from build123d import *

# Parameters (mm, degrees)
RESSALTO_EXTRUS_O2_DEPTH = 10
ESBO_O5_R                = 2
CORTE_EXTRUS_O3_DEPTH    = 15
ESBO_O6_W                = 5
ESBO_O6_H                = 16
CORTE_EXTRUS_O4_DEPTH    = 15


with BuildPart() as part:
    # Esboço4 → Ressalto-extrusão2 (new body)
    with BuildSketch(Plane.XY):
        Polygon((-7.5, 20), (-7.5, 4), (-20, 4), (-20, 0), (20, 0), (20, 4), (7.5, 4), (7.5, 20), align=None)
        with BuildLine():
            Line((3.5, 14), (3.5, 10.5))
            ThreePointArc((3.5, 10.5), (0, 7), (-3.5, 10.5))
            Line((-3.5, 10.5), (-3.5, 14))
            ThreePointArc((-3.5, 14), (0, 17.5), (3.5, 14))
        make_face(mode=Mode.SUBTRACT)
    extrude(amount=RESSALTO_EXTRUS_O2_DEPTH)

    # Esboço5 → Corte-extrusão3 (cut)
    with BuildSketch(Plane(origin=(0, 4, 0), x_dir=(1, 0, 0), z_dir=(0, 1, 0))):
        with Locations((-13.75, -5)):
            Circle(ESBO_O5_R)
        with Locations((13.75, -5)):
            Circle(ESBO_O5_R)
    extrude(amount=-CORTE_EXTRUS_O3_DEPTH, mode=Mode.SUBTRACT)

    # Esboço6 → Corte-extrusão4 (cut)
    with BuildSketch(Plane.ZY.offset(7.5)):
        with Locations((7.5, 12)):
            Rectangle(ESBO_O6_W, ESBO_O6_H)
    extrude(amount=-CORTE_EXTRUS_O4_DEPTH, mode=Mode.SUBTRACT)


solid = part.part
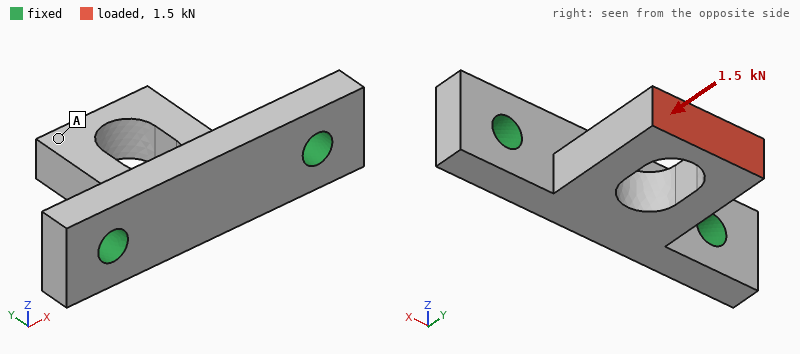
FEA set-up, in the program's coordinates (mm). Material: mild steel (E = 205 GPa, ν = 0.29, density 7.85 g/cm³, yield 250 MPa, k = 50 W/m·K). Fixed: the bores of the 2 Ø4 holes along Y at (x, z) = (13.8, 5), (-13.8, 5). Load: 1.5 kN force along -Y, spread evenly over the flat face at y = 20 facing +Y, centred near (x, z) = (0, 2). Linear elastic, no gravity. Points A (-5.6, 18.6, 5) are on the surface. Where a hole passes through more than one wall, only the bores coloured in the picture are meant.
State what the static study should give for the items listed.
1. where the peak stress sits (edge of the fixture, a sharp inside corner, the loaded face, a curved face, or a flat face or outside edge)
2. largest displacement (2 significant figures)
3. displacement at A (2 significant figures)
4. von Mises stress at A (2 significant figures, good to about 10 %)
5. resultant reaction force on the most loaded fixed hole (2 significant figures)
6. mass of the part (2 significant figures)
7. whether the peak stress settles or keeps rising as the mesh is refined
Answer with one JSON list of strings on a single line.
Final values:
["edge of the fixture", "18 µm", "14 µm", "24 MPa", "780 N", "19 g", "keeps rising"]
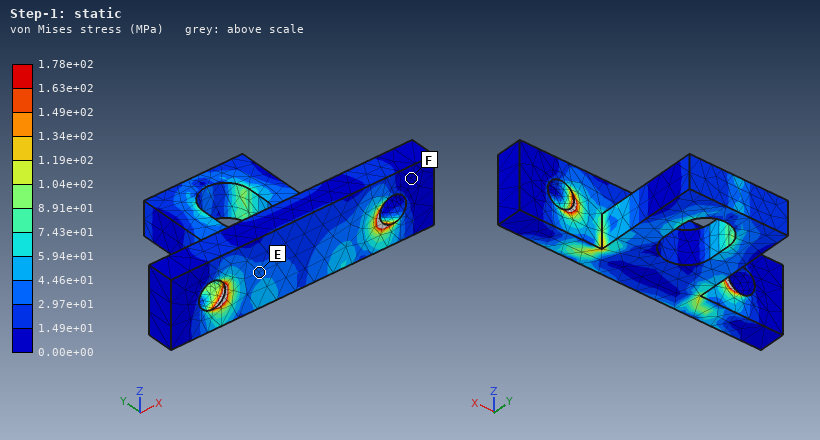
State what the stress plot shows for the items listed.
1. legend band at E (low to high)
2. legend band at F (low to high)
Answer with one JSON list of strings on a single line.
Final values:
["2.97e+01 to 4.46e+01 MPa", "0.00e+00 to 1.49e+01 MPa"]
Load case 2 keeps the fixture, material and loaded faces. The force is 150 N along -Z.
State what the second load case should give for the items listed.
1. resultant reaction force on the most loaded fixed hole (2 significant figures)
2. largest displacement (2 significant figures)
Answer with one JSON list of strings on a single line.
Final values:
["76 N", "26 µm"]
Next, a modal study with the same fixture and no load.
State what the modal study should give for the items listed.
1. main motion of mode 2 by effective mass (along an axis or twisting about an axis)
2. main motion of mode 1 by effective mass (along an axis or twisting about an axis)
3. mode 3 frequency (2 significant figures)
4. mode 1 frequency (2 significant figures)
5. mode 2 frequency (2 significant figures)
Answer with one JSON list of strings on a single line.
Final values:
["along X", "along Z", "22 kHz", "7900 Hz", "17 kHz"]
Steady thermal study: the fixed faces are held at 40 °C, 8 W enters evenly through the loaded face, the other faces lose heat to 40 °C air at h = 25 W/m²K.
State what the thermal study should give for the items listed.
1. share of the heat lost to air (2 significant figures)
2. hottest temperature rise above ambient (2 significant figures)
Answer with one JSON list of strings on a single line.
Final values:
["10 %", "70 K"]
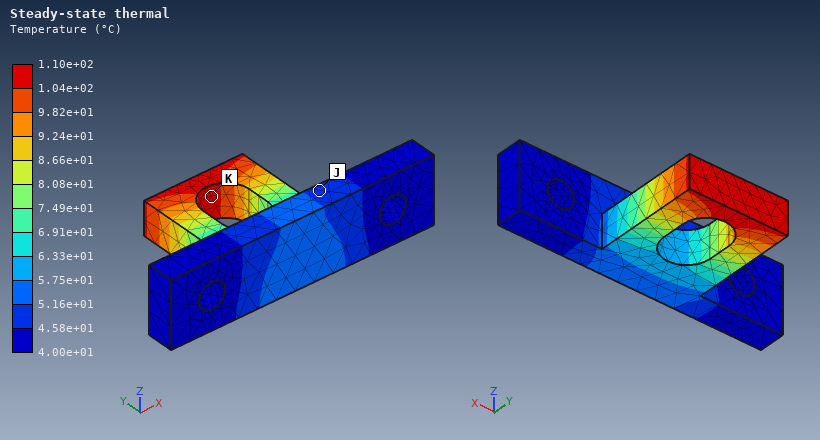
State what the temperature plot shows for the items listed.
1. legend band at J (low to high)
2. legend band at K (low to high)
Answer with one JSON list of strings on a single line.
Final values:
["4.58e+01 to 5.16e+01 °C", "1.04e+02 to 1.10e+02 °C"]
